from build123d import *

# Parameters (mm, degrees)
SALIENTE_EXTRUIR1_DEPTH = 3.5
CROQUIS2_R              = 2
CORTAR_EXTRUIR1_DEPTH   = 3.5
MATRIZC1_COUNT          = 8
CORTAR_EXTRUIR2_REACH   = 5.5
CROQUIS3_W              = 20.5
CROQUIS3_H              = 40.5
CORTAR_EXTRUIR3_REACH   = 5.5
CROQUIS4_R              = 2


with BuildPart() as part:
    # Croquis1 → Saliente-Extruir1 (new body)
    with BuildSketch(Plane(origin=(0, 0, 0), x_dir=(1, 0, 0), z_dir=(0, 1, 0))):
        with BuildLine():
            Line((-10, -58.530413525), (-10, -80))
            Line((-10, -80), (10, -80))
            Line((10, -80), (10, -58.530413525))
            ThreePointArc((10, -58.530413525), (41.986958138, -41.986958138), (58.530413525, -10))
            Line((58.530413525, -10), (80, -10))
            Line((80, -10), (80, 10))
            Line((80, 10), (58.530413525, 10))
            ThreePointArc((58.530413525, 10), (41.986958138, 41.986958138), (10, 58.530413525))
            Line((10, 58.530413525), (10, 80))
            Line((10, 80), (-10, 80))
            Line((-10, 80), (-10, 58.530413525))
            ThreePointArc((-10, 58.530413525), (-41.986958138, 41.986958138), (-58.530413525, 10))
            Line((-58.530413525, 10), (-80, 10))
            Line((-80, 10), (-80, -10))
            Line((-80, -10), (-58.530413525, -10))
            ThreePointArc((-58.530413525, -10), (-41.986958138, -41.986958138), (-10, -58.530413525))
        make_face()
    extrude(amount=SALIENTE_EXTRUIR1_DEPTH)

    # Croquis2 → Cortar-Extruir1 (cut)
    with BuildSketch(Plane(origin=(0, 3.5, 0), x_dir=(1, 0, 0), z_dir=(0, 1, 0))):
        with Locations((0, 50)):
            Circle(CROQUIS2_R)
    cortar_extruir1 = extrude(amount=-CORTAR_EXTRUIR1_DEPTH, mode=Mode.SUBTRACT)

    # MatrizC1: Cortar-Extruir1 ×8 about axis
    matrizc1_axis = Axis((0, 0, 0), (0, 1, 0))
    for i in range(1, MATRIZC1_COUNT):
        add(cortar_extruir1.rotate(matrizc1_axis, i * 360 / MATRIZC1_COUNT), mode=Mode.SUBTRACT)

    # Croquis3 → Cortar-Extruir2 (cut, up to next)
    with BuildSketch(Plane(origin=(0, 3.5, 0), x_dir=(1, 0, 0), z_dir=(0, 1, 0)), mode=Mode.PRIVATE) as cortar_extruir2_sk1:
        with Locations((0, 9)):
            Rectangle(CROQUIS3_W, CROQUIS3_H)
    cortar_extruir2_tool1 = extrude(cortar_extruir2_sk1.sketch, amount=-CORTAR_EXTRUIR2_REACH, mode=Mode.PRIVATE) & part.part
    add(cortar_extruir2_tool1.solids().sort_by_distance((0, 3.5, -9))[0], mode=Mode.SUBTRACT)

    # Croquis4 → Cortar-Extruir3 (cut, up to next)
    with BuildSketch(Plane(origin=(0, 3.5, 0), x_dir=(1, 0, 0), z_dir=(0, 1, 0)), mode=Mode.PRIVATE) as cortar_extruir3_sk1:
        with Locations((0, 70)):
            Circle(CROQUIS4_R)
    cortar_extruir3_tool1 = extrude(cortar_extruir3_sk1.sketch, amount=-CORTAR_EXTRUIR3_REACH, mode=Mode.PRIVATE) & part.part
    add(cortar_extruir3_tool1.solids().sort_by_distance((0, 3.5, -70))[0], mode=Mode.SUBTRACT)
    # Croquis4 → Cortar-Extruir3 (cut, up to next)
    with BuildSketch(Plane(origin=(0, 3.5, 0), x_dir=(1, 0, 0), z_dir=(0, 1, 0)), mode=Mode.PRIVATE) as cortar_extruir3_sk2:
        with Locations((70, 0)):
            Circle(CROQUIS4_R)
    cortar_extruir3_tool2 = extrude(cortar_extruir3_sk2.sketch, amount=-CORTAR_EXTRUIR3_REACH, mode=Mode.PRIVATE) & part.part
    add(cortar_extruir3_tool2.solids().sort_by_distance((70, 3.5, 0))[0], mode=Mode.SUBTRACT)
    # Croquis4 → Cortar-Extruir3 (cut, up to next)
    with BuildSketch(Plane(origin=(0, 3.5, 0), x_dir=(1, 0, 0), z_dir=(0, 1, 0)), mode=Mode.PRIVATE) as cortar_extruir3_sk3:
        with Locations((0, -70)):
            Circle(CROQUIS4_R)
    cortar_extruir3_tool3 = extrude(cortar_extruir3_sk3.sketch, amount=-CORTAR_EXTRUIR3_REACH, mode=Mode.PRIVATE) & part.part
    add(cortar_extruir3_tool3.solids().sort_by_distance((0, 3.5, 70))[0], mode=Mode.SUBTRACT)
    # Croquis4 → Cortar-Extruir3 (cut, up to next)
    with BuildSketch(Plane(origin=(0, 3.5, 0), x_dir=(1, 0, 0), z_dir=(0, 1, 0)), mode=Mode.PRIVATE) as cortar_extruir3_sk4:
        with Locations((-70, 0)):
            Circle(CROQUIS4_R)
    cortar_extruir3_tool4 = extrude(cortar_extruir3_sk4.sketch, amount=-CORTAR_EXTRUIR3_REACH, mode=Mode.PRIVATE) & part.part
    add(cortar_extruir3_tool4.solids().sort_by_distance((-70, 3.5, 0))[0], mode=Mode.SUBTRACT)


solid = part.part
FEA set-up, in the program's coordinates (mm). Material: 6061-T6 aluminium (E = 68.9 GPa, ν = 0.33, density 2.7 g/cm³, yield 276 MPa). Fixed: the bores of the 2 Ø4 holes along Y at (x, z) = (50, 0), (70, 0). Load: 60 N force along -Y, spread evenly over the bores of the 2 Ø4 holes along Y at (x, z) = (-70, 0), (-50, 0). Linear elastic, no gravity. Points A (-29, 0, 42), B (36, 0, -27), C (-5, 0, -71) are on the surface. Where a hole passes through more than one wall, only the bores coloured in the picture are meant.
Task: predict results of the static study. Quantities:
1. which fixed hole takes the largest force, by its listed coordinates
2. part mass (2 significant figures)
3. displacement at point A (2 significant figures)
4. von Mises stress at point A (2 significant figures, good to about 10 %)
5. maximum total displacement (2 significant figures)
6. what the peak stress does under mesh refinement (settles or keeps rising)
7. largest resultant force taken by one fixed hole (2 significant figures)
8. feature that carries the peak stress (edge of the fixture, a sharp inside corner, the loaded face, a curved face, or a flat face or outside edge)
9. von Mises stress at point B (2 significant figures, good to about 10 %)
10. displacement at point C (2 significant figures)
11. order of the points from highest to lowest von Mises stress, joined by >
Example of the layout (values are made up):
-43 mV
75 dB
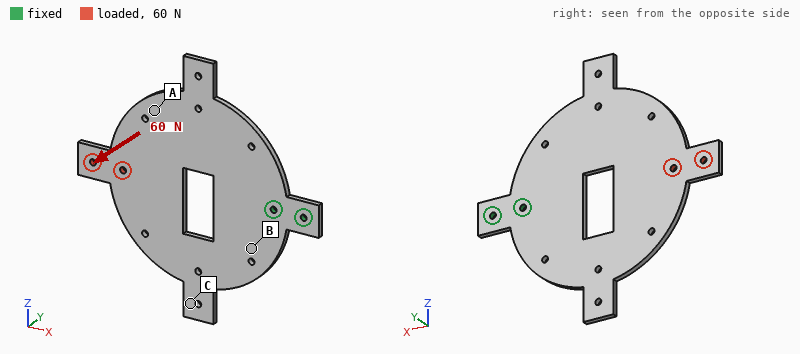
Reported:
(50, 0)
110 g
1.1 mm
13 MPa
2.3 mm
keeps rising
210 N
edge of the fixture
30 MPa
0.58 mm
B > A > C
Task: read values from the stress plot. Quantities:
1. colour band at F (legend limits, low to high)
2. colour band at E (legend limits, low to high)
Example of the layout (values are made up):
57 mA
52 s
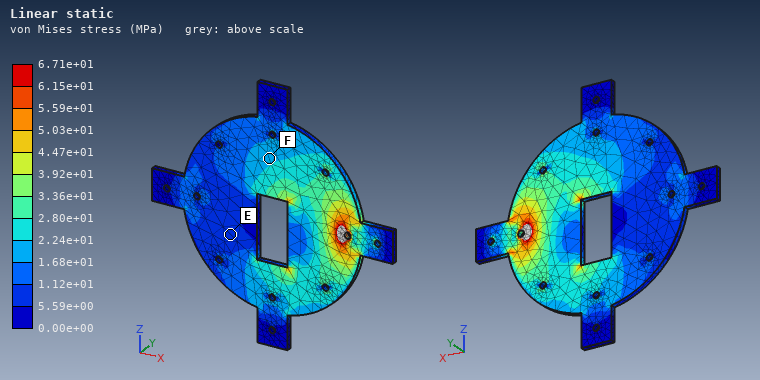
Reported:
1.68e+01 to 2.24e+01 MPa
5.59e+00 to 1.12e+01 MPa
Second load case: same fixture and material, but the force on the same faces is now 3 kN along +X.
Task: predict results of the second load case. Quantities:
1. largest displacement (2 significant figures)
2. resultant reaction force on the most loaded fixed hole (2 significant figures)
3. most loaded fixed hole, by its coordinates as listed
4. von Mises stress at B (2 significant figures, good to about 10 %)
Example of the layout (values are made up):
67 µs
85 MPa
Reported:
56 µm
2.1 kN
(50, 0)
15 MPa
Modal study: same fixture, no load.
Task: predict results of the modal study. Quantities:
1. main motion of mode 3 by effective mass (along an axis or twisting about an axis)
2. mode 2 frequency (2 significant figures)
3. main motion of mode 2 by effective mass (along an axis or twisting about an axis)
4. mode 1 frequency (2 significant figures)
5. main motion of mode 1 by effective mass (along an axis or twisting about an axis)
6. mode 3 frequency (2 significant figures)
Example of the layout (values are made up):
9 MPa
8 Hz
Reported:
along Y
310 Hz
twisting about X
180 Hz
along Y
710 Hz
